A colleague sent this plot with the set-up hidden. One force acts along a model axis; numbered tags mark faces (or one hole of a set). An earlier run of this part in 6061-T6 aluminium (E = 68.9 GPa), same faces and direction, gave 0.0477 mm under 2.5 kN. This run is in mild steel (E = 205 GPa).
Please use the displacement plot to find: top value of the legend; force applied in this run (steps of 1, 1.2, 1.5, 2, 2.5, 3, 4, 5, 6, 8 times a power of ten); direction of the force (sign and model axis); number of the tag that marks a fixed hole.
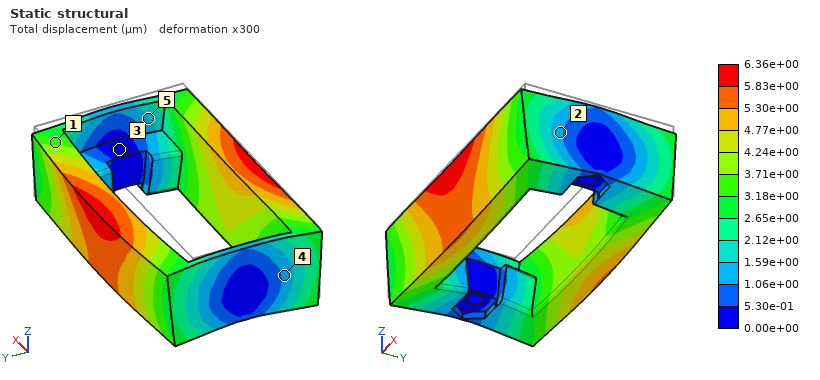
6.36e+00 µm
1 kN
-Z
3
